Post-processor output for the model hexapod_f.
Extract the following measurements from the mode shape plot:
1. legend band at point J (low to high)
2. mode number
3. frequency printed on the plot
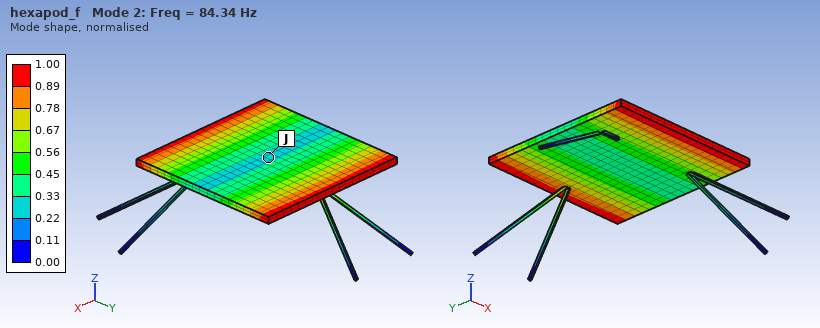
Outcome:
0.22 to 0.33
2
84.34 Hz
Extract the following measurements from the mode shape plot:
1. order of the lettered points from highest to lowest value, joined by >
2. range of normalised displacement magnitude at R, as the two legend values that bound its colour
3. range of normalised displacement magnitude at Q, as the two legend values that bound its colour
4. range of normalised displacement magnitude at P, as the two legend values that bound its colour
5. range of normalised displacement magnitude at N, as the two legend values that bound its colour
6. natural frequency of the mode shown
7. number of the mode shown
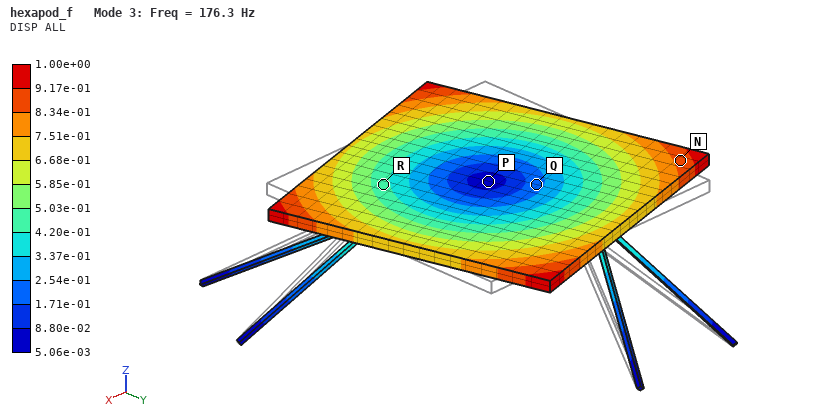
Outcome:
N > R > Q > P
4.20e-01 to 5.03e-01
1.71e-01 to 2.54e-01
5.06e-03 to 8.80e-02
8.34e-01 to 9.17e-01
176.3 Hz
3
